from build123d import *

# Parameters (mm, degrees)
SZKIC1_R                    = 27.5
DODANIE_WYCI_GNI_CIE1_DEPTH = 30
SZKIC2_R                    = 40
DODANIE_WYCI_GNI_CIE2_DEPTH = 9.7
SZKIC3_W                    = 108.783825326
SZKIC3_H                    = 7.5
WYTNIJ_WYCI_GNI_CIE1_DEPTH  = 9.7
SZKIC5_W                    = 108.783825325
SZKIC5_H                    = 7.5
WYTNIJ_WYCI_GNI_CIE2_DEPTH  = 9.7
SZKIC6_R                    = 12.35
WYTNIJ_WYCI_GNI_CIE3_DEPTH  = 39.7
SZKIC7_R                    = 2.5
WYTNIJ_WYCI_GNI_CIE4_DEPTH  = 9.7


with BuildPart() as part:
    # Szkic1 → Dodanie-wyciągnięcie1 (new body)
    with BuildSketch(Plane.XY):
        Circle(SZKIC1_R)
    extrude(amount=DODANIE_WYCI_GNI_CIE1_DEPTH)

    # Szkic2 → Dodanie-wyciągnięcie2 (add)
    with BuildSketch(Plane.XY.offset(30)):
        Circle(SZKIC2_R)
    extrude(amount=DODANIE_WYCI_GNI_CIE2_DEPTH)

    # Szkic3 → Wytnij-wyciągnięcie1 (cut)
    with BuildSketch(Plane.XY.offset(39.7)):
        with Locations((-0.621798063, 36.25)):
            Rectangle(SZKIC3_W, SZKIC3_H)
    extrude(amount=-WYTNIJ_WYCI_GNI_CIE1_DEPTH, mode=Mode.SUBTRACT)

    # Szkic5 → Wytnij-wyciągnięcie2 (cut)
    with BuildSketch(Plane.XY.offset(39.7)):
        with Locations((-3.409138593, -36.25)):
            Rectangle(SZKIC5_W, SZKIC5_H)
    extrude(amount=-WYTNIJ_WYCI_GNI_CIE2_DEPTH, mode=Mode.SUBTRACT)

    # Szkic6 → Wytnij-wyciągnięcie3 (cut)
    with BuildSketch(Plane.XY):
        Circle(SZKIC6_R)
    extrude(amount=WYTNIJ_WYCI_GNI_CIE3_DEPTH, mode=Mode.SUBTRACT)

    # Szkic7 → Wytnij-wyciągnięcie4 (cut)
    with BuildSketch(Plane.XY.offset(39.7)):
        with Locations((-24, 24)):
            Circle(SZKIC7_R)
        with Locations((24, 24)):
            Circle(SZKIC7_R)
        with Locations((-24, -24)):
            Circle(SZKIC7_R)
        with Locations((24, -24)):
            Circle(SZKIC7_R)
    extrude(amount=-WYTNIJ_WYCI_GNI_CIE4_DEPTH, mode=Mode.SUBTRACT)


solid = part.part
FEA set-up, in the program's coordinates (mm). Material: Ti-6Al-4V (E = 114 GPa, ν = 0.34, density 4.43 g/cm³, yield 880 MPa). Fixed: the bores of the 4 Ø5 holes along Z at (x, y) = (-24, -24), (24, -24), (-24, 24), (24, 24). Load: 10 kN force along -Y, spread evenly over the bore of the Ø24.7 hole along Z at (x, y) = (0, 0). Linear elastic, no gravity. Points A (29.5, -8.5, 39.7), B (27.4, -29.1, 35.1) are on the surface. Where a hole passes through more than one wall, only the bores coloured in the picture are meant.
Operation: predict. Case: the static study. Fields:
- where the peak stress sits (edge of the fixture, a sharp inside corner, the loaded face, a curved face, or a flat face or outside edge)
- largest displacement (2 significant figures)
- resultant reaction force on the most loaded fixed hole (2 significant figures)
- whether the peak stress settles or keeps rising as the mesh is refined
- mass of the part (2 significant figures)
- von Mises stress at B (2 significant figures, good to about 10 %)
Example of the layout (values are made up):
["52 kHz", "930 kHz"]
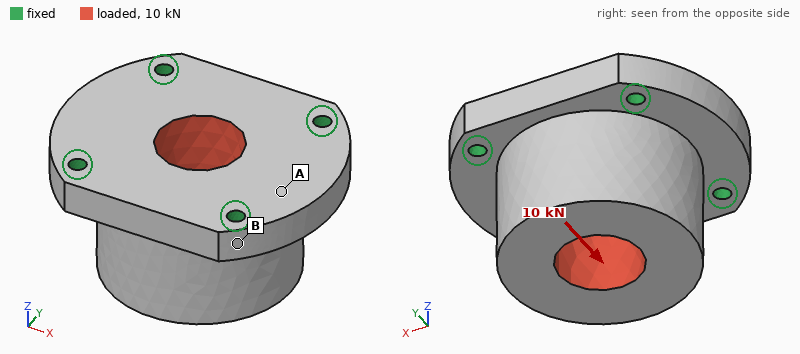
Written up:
["edge of the fixture", "11 µm", "3.1 kN", "keeps rising", "420 g", "13 MPa"]
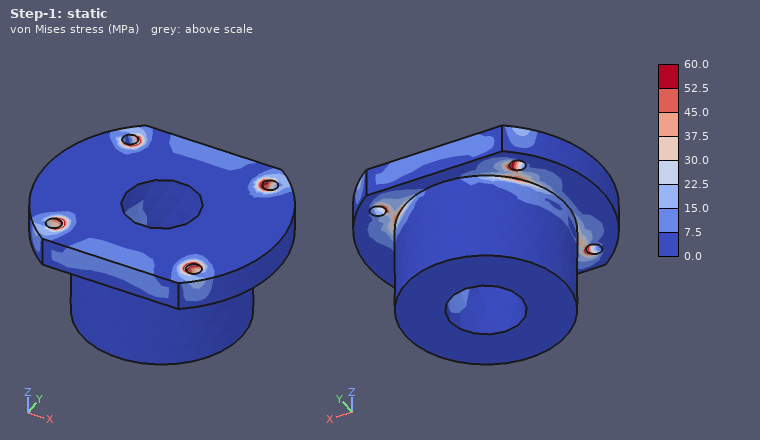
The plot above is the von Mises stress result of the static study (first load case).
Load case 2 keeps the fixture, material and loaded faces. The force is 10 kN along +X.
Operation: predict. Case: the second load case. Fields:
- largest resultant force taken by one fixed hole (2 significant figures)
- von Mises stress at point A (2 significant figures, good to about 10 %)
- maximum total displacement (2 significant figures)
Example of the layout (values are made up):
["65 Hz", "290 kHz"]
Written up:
["3.0 kN", "9.3 MPa", "10 µm"]
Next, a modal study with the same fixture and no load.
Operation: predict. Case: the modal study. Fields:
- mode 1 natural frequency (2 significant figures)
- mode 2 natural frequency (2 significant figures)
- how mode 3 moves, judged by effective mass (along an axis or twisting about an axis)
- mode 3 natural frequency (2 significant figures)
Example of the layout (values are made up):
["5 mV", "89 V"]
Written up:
["9500 Hz", "9600 Hz", "along Z", "11 kHz"]
